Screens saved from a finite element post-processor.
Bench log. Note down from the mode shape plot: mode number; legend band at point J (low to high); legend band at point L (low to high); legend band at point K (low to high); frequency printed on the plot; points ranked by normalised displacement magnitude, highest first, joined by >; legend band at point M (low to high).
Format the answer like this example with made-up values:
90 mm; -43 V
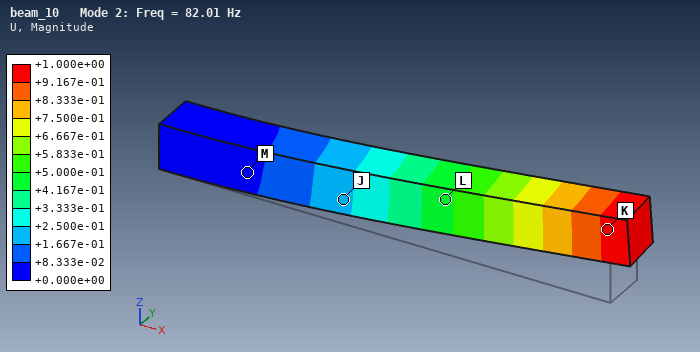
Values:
2; +1.667e-01 to +2.500e-01; +4.167e-01 to +5.000e-01; +9.167e-01 to +1.000e+00; 82.01 Hz; K > L > J > M; +0.000e+00 to +8.333e-02
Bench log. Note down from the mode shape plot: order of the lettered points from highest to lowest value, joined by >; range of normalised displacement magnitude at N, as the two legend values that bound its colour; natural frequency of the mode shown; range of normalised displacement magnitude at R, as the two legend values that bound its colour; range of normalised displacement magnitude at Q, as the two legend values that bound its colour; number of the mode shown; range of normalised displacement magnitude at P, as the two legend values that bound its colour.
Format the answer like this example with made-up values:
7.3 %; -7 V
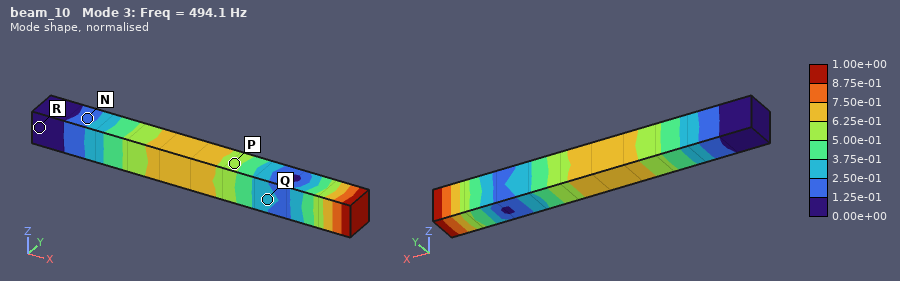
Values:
P > Q > N > R; 1.25e-01 to 2.50e-01; 494.1 Hz; 0.00e+00 to 1.25e-01; 2.50e-01 to 3.75e-01; 3; 5.00e-01 to 6.25e-01
